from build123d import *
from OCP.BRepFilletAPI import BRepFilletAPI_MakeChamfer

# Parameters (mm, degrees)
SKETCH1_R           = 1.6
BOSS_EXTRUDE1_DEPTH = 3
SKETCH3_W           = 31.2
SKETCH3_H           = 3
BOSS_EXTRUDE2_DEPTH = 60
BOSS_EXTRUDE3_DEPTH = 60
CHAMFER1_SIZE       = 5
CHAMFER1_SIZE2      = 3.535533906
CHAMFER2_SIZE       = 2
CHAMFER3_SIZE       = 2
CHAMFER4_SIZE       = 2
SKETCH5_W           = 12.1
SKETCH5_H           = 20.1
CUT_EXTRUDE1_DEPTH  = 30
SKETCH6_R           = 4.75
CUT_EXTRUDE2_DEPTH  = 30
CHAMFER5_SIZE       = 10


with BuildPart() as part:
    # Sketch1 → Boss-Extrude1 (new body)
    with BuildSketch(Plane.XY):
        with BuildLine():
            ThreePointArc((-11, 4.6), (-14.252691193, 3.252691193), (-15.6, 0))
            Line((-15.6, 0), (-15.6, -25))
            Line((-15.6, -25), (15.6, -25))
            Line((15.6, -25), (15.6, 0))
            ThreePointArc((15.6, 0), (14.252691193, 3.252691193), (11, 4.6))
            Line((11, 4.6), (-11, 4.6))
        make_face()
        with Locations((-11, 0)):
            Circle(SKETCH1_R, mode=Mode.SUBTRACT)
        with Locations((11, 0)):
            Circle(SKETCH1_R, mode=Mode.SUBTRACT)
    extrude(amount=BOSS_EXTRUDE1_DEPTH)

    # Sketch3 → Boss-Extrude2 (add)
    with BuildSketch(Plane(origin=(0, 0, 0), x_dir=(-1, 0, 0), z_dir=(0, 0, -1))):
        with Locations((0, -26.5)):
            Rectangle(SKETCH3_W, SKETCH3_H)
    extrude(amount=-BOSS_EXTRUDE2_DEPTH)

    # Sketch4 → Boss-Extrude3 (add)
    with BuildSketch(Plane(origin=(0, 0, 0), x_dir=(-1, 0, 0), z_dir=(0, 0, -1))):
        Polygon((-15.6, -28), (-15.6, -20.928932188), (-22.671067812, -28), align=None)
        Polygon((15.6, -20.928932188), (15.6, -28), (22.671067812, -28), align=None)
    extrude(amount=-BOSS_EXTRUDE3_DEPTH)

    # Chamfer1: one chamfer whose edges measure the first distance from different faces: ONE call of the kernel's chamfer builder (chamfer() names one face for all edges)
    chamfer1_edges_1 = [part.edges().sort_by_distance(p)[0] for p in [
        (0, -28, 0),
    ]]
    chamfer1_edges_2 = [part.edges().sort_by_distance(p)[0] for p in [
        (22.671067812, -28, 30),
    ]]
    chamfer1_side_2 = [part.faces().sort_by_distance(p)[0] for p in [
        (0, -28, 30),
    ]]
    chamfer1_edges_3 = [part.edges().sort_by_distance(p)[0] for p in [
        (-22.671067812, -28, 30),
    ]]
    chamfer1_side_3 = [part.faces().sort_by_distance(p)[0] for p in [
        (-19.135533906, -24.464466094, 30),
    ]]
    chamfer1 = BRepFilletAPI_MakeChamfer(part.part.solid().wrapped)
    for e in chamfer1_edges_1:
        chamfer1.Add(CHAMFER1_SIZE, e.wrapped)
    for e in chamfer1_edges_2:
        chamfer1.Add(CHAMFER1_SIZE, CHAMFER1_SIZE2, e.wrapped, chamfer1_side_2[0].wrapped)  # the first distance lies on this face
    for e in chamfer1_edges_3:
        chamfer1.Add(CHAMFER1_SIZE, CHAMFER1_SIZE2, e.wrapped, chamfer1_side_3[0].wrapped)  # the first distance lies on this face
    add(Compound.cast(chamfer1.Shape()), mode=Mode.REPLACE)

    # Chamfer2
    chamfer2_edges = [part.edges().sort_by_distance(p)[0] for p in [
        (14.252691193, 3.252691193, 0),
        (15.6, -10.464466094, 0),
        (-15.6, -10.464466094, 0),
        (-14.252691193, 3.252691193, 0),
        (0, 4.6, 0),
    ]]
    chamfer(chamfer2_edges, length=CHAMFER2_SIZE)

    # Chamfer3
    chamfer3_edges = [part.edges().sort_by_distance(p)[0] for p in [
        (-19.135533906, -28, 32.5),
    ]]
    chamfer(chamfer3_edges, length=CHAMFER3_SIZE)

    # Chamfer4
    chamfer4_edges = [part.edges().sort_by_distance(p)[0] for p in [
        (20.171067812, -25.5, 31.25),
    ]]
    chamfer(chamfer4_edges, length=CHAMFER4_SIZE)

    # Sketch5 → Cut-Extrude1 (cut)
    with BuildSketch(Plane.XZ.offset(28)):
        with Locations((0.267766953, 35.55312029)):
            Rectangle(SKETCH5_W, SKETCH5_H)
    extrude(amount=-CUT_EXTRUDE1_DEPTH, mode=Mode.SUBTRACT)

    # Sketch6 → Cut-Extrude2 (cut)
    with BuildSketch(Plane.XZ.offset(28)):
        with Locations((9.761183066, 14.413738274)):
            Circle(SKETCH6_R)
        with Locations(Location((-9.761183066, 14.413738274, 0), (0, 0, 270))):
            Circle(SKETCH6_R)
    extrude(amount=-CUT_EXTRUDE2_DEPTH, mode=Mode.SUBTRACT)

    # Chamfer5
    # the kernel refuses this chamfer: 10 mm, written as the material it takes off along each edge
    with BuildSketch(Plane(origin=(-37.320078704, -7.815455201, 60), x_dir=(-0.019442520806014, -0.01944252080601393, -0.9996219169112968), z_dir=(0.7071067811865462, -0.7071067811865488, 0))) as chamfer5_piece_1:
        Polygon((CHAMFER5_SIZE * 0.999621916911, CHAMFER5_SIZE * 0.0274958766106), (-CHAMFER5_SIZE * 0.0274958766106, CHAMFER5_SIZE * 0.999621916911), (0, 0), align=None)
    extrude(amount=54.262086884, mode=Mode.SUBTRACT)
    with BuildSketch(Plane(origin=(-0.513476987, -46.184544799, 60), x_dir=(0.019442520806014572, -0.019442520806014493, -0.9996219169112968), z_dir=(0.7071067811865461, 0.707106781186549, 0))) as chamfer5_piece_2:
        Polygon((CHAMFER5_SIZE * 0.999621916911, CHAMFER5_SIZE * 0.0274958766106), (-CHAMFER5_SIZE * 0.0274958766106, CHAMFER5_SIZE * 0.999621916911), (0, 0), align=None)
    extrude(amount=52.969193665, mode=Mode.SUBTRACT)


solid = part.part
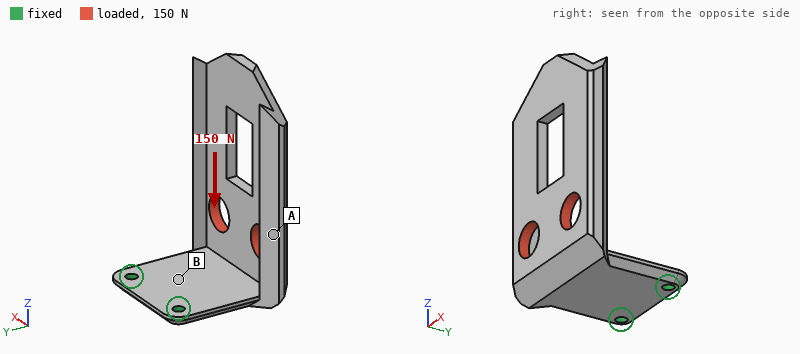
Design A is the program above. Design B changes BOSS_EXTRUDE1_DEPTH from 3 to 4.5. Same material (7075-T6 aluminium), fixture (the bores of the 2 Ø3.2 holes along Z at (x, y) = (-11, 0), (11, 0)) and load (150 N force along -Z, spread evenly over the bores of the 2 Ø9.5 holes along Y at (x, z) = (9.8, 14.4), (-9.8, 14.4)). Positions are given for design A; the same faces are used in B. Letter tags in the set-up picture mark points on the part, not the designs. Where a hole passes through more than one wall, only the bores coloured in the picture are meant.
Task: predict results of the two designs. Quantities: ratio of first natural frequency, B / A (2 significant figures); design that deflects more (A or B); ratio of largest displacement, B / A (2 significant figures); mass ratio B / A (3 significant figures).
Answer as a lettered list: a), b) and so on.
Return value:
a) 1.7
b) A
c) 0.30
d) 1.17
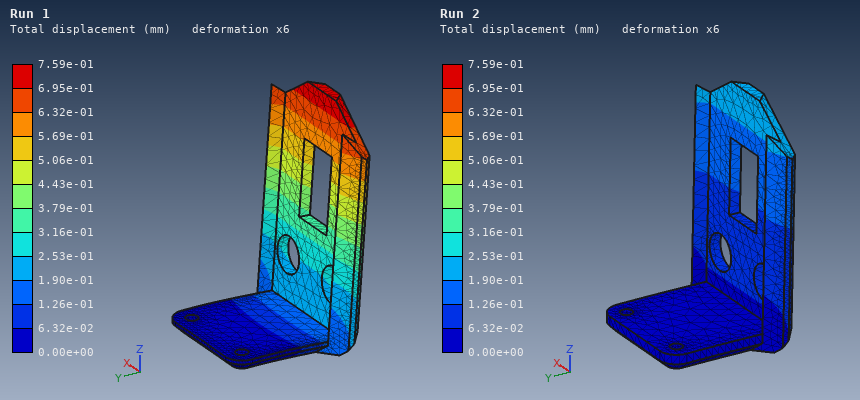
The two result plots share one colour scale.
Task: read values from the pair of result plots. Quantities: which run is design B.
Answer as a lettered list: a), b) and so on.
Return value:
a) Run 2
